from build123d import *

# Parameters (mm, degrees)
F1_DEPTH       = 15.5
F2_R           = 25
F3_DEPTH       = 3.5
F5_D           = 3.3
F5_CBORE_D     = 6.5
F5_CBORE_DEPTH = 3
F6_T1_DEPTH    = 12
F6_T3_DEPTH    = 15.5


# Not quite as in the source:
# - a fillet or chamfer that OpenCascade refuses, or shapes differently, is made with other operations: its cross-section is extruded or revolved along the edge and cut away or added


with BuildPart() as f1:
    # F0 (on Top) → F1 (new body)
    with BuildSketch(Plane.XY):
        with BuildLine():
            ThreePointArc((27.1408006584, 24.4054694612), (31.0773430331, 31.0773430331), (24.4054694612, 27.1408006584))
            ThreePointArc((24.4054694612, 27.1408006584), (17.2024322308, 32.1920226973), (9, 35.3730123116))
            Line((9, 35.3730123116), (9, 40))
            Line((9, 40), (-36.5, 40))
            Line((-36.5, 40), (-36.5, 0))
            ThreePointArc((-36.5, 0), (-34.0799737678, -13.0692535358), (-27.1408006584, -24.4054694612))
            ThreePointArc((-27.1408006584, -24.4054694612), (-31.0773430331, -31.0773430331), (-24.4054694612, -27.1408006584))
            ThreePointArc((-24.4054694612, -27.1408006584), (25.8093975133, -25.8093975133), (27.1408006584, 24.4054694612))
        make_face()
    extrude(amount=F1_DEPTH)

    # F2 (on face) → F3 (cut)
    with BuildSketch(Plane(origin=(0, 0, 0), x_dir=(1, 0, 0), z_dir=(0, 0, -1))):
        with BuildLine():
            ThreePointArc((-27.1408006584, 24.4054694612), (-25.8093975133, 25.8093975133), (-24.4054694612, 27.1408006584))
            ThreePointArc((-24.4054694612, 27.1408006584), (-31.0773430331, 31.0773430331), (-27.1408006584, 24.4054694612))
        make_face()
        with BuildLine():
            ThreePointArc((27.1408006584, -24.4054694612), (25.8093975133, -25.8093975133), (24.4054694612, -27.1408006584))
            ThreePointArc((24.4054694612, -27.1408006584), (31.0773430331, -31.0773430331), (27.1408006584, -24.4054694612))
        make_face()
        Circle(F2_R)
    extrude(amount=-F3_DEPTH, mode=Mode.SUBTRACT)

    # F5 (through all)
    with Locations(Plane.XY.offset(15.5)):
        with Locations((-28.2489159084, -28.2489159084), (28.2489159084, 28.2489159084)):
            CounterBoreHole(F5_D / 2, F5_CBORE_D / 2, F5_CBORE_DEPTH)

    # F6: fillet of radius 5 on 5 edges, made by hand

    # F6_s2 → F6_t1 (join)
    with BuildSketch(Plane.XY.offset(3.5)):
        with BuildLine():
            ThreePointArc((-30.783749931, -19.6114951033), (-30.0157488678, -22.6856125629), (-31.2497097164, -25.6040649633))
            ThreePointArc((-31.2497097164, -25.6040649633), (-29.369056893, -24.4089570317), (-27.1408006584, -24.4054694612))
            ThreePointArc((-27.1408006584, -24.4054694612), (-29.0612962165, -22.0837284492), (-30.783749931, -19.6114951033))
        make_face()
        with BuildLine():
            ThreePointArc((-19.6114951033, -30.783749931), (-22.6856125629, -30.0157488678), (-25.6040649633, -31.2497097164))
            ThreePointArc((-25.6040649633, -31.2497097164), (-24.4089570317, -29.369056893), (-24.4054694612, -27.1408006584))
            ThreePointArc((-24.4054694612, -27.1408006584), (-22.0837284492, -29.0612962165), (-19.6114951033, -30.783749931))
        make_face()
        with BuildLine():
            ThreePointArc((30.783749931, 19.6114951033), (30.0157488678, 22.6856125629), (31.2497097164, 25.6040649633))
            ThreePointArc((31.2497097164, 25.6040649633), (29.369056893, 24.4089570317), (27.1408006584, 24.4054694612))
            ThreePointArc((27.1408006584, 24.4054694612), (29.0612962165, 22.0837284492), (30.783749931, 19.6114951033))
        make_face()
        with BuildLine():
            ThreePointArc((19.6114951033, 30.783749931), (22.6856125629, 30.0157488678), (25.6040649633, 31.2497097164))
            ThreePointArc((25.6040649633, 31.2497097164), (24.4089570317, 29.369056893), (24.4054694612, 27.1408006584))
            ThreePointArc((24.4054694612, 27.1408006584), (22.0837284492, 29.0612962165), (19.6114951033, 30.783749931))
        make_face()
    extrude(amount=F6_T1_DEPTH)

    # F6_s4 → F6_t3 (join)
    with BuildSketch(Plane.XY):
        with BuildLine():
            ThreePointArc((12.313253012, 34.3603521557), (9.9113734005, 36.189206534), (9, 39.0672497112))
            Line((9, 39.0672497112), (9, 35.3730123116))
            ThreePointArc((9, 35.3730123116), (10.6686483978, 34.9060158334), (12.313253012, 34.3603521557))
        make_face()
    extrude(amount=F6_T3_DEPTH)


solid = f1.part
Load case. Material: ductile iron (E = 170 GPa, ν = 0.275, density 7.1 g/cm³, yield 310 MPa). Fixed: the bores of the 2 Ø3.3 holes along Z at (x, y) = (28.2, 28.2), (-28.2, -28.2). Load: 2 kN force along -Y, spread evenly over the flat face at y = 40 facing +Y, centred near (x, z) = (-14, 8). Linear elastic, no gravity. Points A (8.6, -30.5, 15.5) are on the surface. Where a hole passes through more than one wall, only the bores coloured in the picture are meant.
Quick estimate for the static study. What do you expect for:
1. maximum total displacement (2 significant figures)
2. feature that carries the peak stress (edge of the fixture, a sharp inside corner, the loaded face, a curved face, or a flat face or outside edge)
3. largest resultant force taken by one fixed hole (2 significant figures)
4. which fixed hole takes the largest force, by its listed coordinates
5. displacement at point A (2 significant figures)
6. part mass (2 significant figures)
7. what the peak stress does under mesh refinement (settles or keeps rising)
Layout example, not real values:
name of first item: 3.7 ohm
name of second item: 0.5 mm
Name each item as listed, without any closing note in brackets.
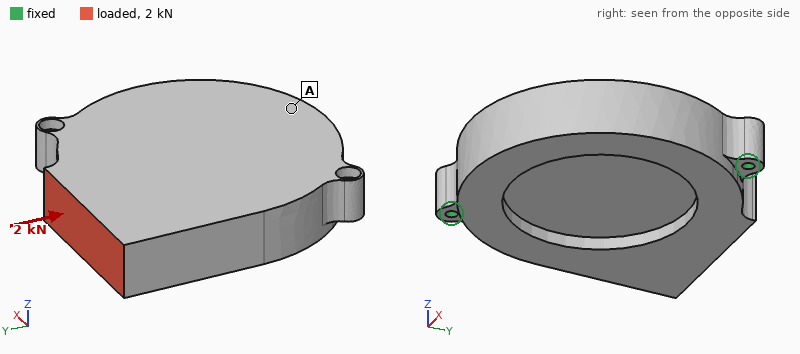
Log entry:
maximum total displacement: 3.1 µm
feature that carries the peak stress: edge of the fixture
largest resultant force taken by one fixed hole: 1.3 kN
which fixed hole takes the largest force, by its listed coordinates: (-28.2, -28.2)
displacement at point A: 1.2 µm
part mass: 470 g
what the peak stress does under mesh refinement: keeps rising
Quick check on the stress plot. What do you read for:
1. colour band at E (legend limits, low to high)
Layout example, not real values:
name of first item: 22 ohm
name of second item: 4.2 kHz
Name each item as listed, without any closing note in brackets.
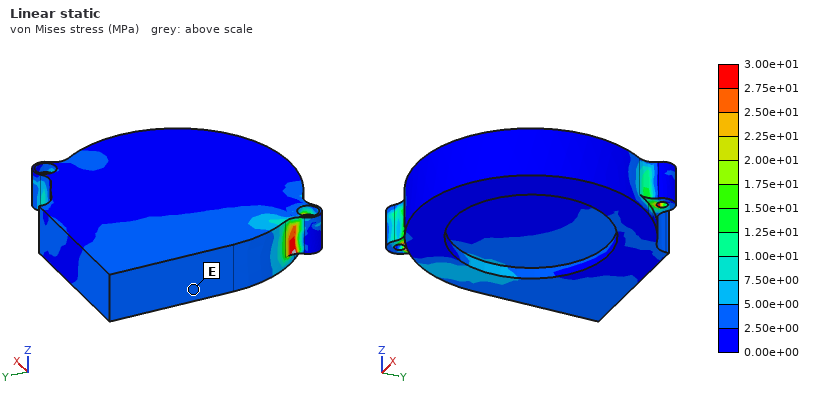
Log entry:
colour band at E: 2.50e+00 to 5.00e+00 MPa
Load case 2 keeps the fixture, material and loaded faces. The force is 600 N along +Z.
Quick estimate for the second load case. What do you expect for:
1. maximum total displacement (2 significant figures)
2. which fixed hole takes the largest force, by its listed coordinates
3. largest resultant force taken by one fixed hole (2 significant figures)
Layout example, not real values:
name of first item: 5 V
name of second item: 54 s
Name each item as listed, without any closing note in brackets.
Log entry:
maximum total displacement: 49 µm
which fixed hole takes the largest force, by its listed coordinates: (28.2, 28.2)
largest resultant force taken by one fixed hole: 460 N
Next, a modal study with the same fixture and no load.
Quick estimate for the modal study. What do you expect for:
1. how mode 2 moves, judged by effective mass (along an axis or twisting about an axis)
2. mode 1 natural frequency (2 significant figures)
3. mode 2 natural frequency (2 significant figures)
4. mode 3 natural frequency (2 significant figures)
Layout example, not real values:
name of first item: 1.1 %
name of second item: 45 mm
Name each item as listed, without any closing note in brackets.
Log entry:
how mode 2 moves, judged by effective mass: along Z
mode 1 natural frequency: 1800 Hz
mode 2 natural frequency: 4000 Hz
mode 3 natural frequency: 8600 Hz
